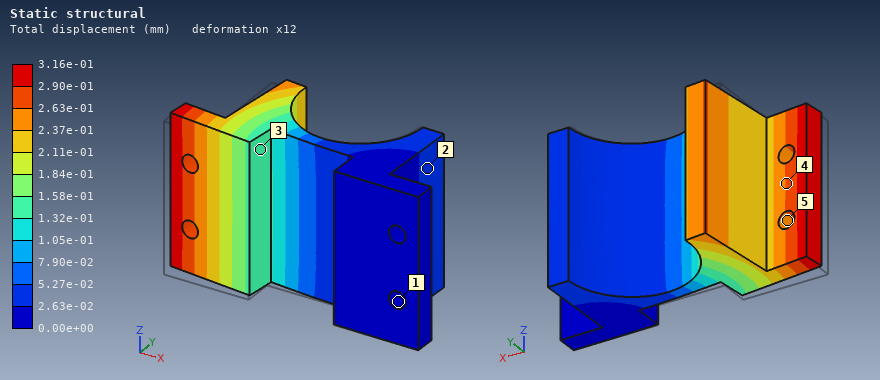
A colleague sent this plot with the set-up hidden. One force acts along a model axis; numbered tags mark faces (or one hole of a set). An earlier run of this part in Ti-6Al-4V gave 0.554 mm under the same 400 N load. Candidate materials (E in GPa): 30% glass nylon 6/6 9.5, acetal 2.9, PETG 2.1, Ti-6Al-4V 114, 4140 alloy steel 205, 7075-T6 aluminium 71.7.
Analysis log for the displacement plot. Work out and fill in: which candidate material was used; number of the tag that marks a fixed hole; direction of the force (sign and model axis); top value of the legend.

4140 alloy steel
1
+Y
3.16e-01 mm
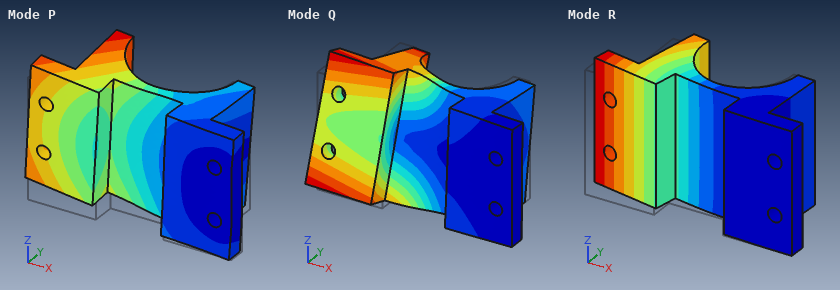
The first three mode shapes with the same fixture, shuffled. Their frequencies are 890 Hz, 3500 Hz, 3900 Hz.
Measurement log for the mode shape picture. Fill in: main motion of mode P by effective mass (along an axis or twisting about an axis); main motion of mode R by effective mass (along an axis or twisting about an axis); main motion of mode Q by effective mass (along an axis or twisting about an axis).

along Z
along Y
twisting about X
